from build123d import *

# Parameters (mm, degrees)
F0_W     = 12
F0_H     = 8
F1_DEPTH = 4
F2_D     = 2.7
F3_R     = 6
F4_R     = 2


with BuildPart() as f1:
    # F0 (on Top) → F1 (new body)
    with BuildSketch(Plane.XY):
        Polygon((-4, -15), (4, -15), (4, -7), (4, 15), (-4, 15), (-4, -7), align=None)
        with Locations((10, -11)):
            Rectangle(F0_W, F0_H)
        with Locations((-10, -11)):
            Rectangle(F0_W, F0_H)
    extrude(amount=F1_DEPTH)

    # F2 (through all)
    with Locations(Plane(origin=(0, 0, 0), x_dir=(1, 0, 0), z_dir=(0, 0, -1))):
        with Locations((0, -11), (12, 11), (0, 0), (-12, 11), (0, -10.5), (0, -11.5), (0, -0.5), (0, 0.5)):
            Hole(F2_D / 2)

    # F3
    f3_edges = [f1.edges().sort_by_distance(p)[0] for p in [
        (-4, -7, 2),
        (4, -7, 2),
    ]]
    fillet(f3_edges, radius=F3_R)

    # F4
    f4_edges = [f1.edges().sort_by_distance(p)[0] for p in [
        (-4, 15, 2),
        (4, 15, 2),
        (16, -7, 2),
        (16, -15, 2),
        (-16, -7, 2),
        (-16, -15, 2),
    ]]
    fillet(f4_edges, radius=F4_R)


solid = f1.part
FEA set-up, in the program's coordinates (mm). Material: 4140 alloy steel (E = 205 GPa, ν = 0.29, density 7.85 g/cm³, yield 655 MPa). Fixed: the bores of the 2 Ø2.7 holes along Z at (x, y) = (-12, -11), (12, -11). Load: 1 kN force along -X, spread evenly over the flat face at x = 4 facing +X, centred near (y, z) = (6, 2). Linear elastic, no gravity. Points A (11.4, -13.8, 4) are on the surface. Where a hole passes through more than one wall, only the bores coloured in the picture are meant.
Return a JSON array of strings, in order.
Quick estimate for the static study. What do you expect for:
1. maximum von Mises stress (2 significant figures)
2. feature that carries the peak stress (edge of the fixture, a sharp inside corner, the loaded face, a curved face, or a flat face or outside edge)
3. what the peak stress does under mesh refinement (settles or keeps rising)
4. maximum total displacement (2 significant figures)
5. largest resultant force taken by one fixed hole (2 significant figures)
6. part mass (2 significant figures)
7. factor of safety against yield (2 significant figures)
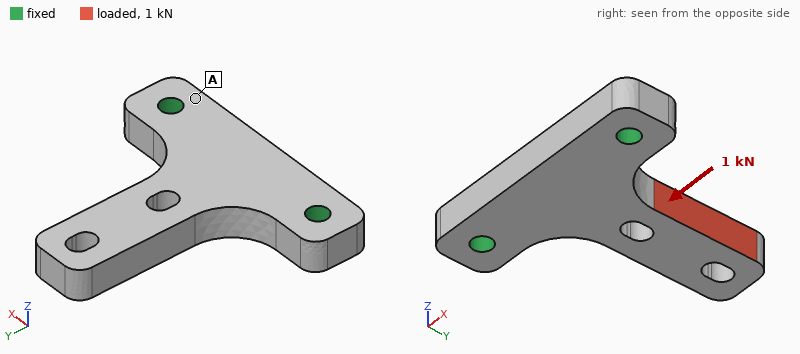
["290 MPa", "a curved face", "settles", "51 µm", "930 N", "13 g", "2.2"]
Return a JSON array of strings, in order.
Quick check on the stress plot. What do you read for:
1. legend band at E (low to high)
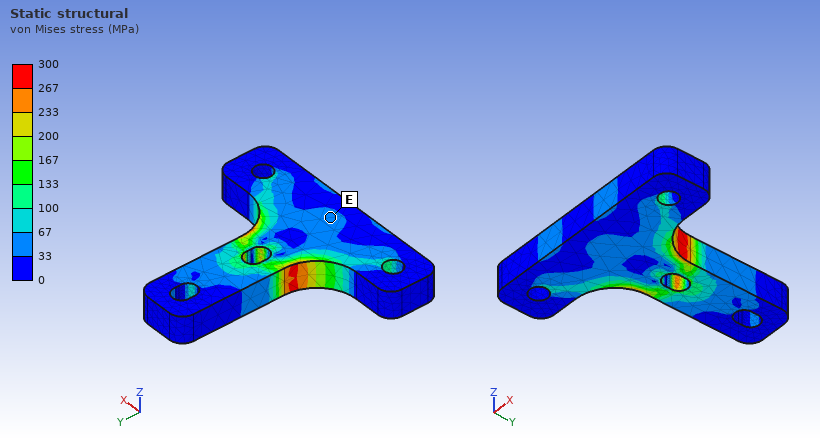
["33 to 67 MPa"]
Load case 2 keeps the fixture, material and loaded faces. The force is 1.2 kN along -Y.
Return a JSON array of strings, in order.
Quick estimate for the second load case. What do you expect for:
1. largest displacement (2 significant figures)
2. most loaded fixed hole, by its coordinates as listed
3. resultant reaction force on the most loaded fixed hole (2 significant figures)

["28 µm", "(12, -11)", "870 N"]
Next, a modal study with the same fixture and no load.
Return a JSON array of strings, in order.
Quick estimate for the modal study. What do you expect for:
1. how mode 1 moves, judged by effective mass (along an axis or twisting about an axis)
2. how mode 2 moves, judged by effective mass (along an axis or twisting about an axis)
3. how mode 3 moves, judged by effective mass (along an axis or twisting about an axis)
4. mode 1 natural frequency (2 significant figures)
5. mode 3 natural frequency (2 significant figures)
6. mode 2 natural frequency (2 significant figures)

["along Z", "along X", "along Z", "4800 Hz", "23 kHz", "13 kHz"]
